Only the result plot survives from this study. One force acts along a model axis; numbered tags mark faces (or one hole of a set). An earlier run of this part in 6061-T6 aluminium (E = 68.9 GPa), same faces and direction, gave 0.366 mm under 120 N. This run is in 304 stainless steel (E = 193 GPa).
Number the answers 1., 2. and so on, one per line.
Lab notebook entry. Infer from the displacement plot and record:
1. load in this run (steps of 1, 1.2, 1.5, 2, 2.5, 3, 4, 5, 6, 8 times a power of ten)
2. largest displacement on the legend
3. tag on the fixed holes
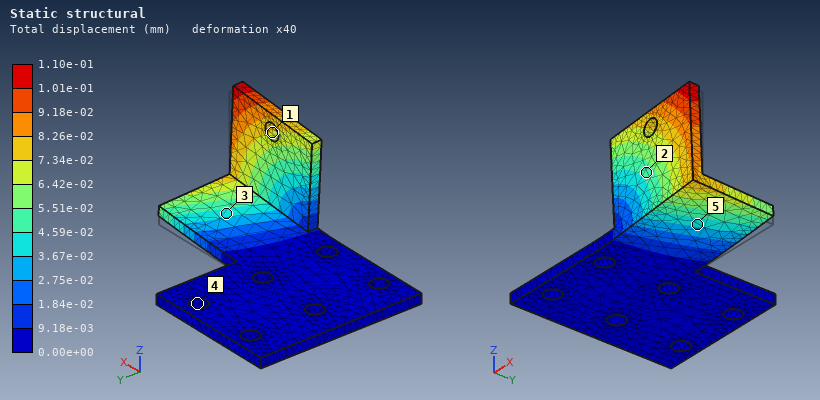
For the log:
1. 100 N
2. 1.10e-01 mm
3. 4
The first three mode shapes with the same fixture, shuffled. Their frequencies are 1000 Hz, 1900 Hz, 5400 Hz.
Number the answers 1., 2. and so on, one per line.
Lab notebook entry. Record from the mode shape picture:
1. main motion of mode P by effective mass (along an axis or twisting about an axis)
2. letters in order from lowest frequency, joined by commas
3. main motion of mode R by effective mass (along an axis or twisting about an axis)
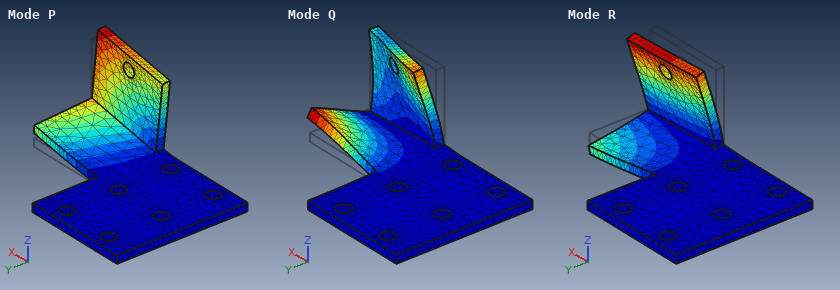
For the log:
1. along Z
2. P, R, Q
3. along Y
